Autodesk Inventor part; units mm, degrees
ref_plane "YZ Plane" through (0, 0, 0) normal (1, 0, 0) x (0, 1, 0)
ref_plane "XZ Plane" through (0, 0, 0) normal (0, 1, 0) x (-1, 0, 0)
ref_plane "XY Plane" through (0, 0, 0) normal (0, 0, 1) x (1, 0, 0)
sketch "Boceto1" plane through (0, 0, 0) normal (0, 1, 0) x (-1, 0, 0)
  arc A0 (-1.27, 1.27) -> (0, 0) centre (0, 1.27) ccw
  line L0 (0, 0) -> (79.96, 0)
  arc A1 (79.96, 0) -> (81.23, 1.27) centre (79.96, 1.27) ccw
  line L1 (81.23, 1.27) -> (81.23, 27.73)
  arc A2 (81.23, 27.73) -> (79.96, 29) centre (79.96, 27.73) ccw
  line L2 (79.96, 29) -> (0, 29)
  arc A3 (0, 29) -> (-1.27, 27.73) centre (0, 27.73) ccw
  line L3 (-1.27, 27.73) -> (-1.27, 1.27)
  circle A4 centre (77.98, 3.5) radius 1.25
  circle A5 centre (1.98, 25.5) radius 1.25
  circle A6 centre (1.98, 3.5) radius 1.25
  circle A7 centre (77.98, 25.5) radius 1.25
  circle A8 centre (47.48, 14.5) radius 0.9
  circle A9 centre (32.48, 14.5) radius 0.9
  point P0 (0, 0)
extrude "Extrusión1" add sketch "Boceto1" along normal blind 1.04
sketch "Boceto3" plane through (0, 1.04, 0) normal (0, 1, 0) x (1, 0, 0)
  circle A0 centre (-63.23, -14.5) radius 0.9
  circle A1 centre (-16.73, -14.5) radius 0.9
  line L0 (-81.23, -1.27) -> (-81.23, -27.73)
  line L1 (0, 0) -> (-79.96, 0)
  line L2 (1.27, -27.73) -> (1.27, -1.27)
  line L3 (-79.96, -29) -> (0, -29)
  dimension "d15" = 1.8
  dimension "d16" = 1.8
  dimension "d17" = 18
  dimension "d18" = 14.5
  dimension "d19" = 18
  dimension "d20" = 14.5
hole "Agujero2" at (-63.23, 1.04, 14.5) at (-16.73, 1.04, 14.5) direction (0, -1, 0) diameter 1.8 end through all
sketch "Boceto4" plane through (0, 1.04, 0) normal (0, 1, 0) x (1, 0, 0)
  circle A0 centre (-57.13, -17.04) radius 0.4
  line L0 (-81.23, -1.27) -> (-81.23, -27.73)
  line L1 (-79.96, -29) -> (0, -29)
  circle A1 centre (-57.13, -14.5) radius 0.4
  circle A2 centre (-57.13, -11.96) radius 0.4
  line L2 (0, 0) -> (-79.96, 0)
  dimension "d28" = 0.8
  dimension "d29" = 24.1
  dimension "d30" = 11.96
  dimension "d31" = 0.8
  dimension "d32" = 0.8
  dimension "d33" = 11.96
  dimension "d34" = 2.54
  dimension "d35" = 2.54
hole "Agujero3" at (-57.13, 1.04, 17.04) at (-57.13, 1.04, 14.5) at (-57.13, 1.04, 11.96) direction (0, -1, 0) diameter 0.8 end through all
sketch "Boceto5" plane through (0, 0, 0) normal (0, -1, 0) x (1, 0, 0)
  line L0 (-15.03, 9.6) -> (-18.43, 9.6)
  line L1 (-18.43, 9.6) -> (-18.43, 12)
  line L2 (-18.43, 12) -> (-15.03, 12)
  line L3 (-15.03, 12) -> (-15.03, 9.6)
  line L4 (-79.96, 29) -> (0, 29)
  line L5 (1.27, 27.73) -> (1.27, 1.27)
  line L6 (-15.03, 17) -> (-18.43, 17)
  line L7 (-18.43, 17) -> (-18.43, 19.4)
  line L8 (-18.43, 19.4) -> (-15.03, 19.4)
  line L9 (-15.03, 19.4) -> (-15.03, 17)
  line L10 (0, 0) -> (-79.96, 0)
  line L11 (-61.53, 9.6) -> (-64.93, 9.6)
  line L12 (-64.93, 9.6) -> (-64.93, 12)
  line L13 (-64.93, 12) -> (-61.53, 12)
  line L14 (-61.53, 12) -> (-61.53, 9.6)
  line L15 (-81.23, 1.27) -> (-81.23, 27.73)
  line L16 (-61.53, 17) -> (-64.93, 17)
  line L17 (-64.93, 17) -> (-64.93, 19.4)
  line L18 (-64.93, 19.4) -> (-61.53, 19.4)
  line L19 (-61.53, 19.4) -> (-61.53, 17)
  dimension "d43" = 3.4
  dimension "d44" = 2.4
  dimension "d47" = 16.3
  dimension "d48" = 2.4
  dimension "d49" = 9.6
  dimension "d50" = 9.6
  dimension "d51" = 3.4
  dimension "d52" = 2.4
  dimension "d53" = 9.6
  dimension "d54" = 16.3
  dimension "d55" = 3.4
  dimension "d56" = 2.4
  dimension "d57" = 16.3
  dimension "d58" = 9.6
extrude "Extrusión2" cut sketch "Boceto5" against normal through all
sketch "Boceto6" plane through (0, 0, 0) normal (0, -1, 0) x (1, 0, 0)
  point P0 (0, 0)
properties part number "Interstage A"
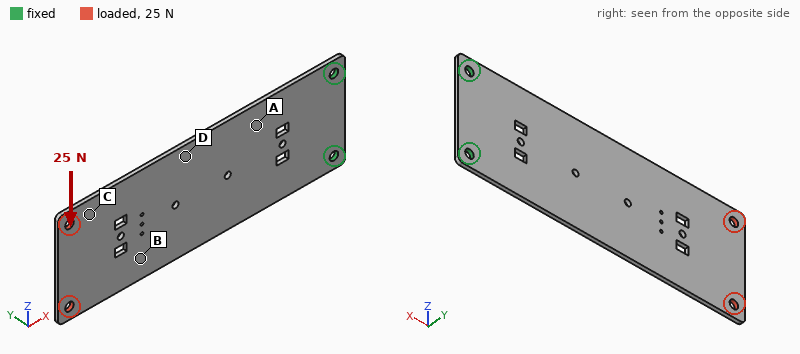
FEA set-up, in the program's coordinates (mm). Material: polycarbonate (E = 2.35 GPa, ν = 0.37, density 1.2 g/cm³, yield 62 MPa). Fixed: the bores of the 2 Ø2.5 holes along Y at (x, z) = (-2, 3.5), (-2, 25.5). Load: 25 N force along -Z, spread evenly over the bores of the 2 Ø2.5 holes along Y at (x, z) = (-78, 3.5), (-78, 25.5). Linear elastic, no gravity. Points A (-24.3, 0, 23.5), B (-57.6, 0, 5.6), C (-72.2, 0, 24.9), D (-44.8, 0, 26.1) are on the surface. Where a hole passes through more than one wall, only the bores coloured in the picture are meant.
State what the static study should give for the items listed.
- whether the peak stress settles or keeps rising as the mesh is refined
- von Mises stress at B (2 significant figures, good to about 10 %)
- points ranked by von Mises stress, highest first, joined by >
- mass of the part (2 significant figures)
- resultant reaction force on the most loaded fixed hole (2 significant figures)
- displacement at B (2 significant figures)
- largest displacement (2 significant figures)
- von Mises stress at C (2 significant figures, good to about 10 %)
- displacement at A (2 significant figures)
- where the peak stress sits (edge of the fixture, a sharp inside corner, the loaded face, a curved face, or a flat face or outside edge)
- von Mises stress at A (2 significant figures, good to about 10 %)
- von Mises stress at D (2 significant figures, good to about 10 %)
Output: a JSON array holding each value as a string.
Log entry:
["keeps rising", "2.4 MPa", "A > D > B > C", "2.9 g", "85 N", "0.55 mm", "0.94 mm", "1.2 MPa", "0.14 mm", "edge of the fixture", "6.0 MPa", "4.7 MPa"]
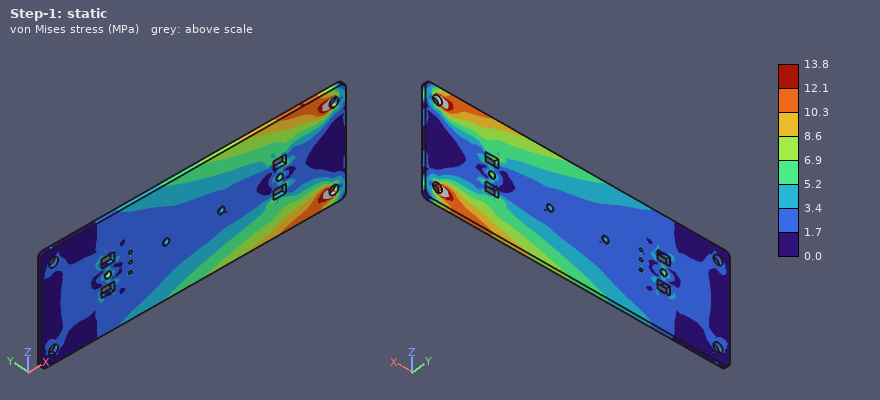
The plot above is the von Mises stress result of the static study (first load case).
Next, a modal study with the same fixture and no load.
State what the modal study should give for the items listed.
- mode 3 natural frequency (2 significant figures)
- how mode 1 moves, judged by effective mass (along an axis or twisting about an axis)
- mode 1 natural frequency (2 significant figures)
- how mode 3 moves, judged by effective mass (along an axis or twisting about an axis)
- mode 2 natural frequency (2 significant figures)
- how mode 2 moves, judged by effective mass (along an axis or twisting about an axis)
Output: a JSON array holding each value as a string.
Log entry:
["230 Hz", "along Y", "37 Hz", "along Y", "210 Hz", "twisting about X"]
